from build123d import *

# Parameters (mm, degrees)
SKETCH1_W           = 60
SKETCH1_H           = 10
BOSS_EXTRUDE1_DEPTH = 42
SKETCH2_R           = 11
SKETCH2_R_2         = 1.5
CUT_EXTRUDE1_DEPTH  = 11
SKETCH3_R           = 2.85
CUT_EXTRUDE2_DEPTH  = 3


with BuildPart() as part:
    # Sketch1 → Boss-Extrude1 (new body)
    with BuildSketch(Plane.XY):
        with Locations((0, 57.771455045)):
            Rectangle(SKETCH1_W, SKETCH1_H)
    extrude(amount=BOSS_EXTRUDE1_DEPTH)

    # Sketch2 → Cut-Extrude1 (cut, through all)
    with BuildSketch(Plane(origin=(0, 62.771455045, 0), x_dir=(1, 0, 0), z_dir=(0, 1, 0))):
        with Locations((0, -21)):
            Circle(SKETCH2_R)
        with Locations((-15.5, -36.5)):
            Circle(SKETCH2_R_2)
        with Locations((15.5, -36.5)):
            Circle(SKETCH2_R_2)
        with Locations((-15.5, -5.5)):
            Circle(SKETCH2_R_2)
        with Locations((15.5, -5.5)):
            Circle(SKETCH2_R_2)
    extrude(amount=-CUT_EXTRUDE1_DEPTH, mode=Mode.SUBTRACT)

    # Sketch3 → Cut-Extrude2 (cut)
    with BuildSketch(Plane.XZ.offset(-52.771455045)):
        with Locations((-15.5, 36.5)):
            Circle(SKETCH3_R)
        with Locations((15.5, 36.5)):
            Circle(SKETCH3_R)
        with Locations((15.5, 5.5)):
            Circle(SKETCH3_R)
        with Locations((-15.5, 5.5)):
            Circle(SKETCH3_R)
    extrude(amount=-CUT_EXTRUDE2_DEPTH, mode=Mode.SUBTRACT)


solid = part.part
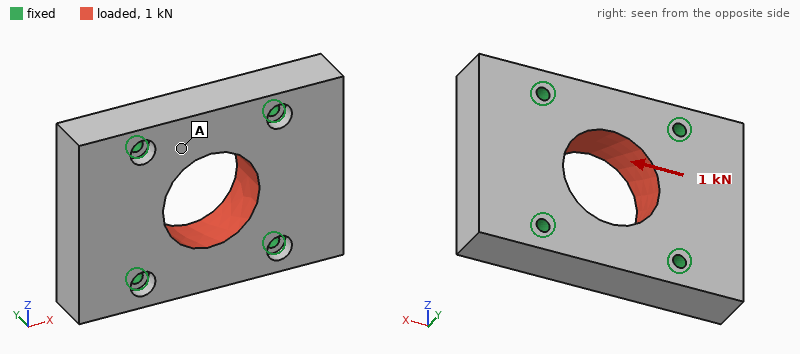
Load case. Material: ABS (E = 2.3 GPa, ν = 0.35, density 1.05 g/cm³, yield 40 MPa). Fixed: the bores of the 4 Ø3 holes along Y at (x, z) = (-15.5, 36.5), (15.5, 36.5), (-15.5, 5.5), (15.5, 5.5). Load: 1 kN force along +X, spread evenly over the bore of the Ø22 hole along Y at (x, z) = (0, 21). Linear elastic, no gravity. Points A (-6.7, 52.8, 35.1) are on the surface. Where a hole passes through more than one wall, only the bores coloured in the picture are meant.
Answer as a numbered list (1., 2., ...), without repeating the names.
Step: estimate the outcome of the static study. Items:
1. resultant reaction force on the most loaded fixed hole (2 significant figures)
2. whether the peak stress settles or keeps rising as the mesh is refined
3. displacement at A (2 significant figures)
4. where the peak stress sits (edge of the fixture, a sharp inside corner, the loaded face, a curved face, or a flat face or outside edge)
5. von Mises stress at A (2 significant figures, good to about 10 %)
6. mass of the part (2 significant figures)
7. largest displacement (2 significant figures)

1. 250 N
2. keeps rising
3. 9.4 µm
4. edge of the fixture
5. 1.3 MPa
6. 22 g
7. 24 µm
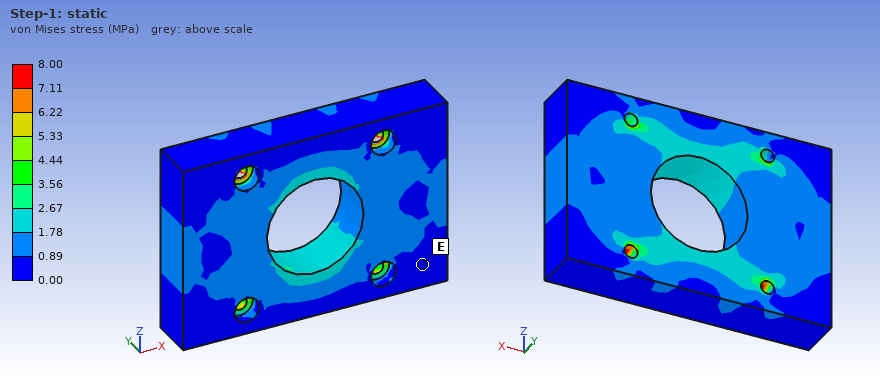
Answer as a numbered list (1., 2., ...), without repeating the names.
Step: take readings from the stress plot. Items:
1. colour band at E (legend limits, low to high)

1. 0.00 to 0.89 MPa
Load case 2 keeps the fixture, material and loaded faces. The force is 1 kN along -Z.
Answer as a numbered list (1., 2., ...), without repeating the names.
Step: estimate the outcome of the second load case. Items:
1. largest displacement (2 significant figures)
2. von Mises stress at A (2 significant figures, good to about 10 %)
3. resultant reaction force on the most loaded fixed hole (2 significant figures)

1. 33 µm
2. 2.2 MPa
3. 260 N
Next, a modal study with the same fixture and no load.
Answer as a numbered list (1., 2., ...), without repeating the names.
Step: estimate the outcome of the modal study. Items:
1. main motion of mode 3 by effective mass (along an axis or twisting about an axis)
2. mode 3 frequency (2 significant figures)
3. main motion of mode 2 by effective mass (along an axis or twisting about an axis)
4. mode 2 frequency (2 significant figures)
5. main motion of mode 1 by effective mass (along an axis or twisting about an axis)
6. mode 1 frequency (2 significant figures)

1. along Y
2. 7800 Hz
3. twisting about Z
4. 5100 Hz
5. along Y
6. 4800 Hz
